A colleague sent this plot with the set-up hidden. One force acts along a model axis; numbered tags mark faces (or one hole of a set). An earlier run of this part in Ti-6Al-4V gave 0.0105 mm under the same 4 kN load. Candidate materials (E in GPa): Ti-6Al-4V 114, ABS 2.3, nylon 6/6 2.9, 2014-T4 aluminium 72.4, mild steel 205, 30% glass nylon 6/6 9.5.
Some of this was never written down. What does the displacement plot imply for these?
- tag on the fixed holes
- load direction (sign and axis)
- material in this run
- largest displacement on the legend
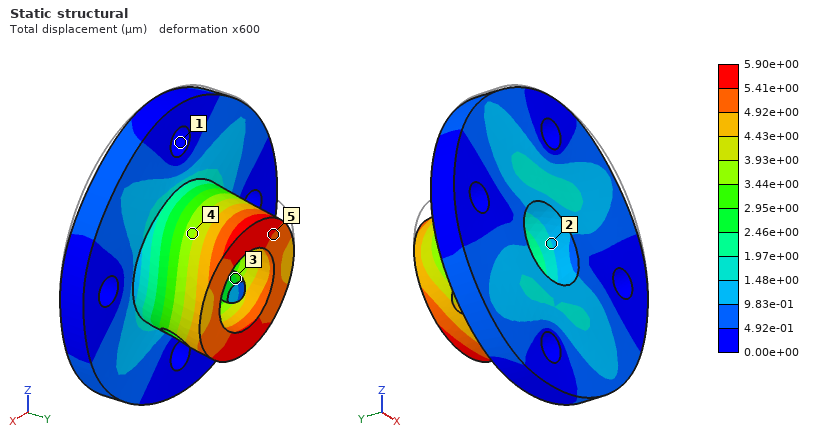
1
-Z
mild steel
5.90e+00 µm
